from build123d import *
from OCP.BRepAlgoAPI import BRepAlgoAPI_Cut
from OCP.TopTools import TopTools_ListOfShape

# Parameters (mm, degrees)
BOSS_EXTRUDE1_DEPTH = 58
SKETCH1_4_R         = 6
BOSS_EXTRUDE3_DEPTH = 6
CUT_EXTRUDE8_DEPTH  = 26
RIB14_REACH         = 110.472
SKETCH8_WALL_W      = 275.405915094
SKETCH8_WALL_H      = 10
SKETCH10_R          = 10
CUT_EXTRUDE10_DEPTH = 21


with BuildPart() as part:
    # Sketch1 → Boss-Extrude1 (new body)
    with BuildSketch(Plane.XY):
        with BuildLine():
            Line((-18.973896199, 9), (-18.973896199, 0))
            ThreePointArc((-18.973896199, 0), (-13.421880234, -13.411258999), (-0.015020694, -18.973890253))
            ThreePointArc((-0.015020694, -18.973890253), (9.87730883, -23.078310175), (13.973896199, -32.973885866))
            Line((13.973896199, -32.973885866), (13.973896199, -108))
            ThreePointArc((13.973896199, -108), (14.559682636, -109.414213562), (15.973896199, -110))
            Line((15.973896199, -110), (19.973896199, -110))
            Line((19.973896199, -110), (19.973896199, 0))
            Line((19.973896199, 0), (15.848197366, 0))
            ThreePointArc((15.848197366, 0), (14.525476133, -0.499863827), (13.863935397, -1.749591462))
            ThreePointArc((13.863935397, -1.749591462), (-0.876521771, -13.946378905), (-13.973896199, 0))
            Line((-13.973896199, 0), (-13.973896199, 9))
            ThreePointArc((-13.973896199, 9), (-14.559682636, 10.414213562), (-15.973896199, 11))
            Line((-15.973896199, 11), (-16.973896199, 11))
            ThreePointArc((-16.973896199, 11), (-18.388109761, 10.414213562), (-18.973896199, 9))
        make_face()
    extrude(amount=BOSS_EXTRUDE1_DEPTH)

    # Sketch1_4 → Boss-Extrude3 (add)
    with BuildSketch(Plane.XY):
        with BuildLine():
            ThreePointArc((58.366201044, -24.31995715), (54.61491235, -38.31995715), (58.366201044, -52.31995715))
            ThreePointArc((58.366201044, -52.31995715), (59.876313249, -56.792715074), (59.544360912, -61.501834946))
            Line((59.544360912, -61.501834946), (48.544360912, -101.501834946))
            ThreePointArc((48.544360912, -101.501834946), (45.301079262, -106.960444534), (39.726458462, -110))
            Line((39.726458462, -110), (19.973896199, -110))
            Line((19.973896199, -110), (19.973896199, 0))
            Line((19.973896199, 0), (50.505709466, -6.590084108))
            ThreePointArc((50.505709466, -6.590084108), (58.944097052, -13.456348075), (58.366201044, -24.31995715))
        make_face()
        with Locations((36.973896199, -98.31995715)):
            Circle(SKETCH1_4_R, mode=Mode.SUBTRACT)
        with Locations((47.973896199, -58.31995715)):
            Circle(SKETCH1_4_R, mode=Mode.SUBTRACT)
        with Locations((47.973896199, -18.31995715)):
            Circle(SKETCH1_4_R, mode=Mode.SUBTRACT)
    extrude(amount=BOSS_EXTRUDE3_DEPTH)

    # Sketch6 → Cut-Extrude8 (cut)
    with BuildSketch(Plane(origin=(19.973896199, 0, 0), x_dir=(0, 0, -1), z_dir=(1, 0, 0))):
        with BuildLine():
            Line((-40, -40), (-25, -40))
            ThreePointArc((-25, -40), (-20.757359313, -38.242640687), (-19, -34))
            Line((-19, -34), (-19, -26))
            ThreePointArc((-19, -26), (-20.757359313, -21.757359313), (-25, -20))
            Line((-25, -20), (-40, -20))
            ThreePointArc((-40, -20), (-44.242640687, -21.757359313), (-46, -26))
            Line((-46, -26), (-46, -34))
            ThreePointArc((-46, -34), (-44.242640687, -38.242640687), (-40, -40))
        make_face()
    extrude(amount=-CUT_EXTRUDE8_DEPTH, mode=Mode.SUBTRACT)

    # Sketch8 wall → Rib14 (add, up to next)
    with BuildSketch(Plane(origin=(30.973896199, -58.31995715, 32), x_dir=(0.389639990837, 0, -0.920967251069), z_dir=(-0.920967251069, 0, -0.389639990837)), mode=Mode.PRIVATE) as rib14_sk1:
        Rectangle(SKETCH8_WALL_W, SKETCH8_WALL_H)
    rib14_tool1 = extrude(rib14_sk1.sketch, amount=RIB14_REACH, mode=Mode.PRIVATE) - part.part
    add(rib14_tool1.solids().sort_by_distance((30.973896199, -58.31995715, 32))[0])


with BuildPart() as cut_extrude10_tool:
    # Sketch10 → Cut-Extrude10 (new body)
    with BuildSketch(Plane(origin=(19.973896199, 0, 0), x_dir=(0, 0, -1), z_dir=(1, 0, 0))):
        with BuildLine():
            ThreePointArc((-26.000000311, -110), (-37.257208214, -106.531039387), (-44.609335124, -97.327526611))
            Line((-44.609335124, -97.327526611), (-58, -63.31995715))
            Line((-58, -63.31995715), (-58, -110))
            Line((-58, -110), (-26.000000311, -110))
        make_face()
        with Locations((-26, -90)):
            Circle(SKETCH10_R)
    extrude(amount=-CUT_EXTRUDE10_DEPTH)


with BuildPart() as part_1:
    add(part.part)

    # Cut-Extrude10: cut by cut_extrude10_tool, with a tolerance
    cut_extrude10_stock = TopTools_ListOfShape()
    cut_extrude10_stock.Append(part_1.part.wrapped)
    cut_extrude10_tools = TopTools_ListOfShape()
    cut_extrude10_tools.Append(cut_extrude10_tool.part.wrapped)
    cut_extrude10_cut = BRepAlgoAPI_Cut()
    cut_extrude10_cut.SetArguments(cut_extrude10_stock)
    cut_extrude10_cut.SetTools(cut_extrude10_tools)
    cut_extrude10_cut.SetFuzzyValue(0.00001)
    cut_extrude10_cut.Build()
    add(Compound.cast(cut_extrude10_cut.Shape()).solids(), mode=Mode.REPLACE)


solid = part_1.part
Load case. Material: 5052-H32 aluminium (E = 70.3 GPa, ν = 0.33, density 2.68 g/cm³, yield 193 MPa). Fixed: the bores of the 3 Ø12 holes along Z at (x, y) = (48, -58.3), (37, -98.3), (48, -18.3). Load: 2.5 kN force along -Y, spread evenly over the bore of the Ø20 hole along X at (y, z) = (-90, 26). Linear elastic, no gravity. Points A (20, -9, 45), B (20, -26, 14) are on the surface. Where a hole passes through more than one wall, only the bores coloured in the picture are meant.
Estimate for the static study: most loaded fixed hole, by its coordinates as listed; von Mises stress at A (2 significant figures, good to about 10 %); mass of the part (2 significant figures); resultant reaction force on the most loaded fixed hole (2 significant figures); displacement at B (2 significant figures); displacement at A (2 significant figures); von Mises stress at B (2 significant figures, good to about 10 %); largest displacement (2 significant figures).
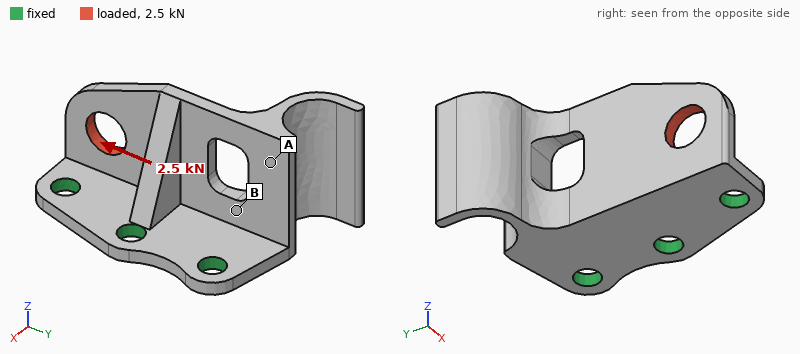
(37, -98.3)
3.9 MPa
200 g
1.5 kN
0.037 mm
0.080 mm
10 MPa
0.13 mm
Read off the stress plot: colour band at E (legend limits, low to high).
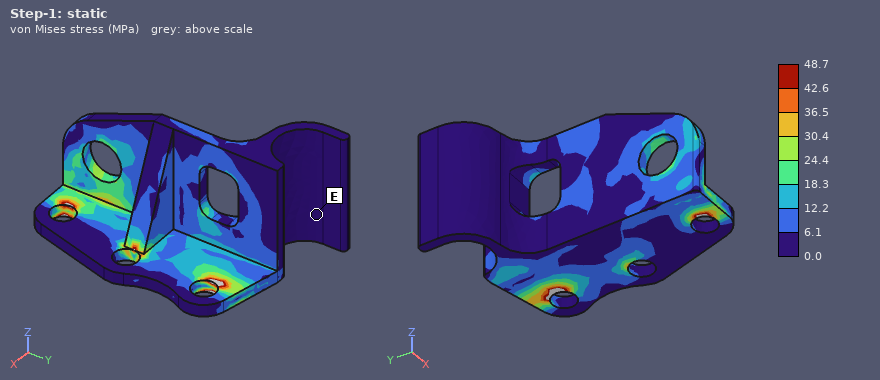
0.0 to 6.1 MPa
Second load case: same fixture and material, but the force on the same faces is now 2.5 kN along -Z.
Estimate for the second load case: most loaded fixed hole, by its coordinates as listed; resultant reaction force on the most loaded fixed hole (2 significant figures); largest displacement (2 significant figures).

(37, -98.3)
2.2 kN
0.15 mm
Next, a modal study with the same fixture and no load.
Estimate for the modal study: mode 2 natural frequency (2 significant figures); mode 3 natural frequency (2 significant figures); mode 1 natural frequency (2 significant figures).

2000 Hz
3000 Hz
920 Hz
